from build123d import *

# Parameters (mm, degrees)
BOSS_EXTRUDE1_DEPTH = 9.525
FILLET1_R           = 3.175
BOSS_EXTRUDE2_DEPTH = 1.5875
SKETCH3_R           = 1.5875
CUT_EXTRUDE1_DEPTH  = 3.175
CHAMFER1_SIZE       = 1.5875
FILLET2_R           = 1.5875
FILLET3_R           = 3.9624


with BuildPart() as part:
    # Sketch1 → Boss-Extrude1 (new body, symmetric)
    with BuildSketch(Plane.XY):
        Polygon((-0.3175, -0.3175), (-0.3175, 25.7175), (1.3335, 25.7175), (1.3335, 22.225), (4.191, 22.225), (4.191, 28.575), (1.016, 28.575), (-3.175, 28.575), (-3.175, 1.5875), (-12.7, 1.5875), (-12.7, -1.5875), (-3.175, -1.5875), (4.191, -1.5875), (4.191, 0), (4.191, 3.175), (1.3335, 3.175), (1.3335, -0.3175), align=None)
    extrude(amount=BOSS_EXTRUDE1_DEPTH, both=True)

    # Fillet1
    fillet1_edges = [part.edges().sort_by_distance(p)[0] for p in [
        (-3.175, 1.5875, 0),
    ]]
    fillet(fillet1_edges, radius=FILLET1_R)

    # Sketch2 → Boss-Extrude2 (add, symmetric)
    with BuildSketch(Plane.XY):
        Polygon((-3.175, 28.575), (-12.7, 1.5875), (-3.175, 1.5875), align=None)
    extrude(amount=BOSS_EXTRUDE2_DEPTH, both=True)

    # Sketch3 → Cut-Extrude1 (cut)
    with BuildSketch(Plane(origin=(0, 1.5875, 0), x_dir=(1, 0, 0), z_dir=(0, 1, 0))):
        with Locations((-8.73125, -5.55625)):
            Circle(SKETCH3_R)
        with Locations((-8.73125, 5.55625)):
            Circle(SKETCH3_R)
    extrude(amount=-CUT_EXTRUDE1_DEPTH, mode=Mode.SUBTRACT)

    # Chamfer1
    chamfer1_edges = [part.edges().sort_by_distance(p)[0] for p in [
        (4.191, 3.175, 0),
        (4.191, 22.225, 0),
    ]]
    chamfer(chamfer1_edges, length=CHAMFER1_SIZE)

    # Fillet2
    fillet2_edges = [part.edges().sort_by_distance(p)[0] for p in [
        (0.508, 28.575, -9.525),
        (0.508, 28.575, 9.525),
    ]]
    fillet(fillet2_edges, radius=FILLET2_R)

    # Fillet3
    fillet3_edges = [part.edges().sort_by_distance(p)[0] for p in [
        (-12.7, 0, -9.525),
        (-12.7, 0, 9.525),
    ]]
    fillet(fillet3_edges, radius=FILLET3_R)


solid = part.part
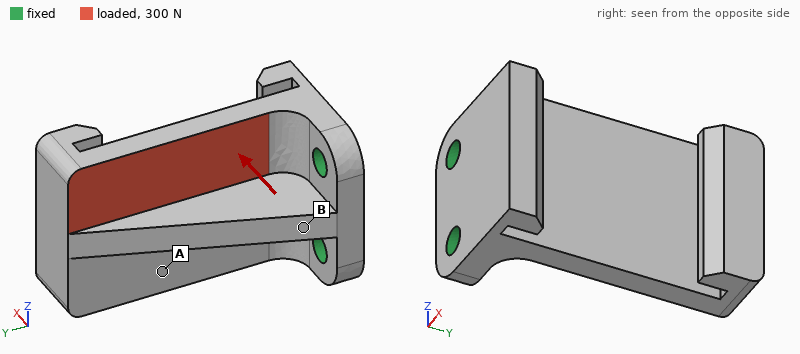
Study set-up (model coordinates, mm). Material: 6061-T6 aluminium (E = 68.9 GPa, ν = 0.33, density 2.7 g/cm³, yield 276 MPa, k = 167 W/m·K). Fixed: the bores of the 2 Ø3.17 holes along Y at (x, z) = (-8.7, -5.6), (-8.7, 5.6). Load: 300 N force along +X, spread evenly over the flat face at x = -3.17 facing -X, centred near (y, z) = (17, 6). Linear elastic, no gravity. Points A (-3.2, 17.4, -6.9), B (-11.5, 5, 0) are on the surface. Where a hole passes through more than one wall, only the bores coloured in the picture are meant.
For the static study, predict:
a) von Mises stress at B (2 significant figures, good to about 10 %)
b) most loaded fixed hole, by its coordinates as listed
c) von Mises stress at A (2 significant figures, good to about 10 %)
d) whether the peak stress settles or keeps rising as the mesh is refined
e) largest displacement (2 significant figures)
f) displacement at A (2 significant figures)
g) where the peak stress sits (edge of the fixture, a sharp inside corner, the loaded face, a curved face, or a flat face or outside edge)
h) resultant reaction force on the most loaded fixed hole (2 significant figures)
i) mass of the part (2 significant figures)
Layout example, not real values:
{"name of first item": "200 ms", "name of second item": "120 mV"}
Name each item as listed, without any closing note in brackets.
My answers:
{"von Mises stress at B": "57 MPa", "most loaded fixed hole, by its coordinates as listed": "(-8.7, 5.6)", "von Mises stress at A": "18 MPa", "whether the peak stress settles or keeps rising as the mesh is refined": "keeps rising", "largest displacement": "0.14 mm", "displacement at A": "0.041 mm", "where the peak stress sits": "edge of the fixture", "resultant reaction force on the most loaded fixed hole": "280 N", "mass of the part": "8.8 g"}
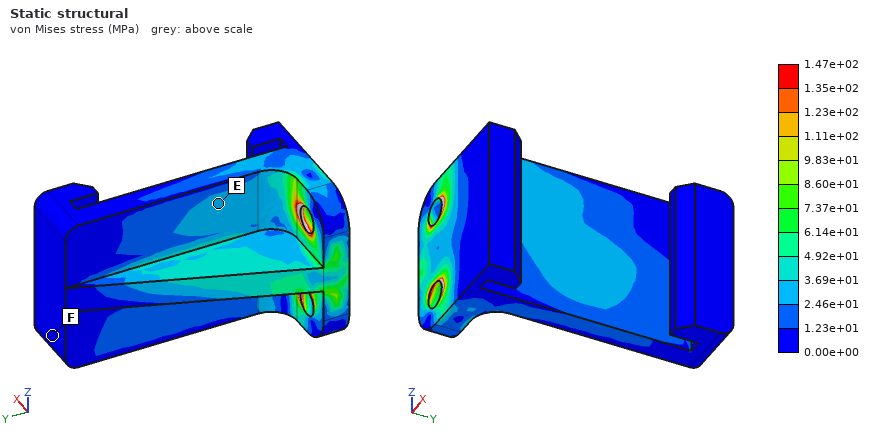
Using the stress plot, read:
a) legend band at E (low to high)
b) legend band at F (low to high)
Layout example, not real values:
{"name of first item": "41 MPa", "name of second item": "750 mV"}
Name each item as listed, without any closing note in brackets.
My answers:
{"legend band at E": "2.46e+01 to 3.69e+01 MPa", "legend band at F": "0.00e+00 to 1.23e+01 MPa"}
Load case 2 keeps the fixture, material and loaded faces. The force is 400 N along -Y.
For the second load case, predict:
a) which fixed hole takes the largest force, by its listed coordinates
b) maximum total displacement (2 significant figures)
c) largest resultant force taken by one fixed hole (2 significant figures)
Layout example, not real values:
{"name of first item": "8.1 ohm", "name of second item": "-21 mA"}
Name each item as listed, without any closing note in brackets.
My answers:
{"which fixed hole takes the largest force, by its listed coordinates": "(-8.7, 5.6)", "maximum total displacement": "35 µm", "largest resultant force taken by one fixed hole": "380 N"}
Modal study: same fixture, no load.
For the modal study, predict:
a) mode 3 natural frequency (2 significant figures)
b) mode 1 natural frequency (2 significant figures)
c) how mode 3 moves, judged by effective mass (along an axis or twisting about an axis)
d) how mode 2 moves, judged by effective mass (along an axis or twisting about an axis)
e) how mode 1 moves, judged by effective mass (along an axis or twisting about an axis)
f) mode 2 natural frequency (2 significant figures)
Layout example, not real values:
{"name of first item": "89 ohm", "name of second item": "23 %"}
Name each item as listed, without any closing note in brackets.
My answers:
{"mode 3 natural frequency": "8200 Hz", "mode 1 natural frequency": "3900 Hz", "how mode 3 moves, judged by effective mass": "twisting about Y", "how mode 2 moves, judged by effective mass": "along Z", "how mode 1 moves, judged by effective mass": "along X", "mode 2 natural frequency": "6000 Hz"}
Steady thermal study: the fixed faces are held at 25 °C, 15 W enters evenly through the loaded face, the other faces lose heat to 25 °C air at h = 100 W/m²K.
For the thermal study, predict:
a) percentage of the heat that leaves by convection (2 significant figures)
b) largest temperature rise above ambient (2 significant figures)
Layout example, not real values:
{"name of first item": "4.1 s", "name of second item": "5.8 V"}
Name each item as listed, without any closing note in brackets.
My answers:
{"percentage of the heat that leaves by convection": "18 %", "largest temperature rise above ambient": "23 K"}
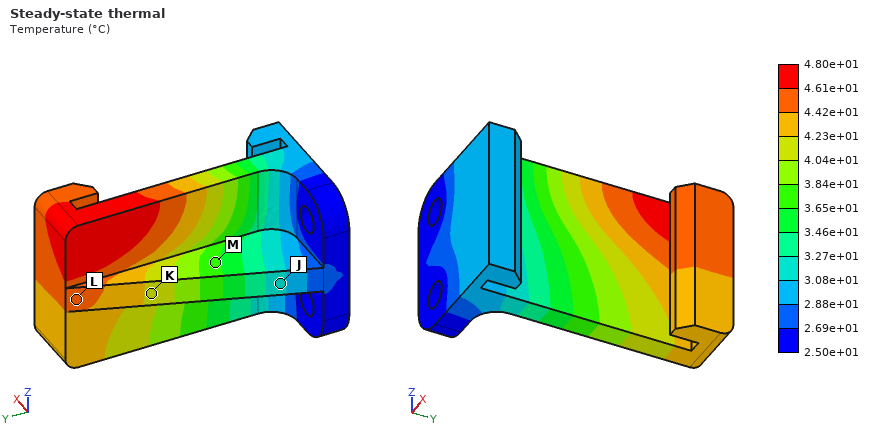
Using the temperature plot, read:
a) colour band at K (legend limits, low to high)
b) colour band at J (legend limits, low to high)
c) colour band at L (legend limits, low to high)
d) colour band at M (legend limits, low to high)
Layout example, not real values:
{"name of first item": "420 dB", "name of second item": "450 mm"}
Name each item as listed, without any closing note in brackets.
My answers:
{"colour band at K": "4.04e+01 to 4.23e+01 °C", "colour band at J": "3.08e+01 to 3.27e+01 °C", "colour band at L": "4.42e+01 to 4.61e+01 °C", "colour band at M": "3.65e+01 to 3.84e+01 °C"}
